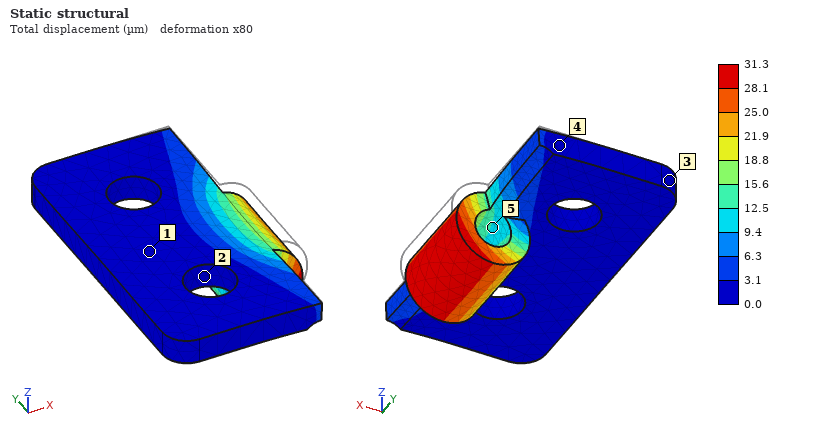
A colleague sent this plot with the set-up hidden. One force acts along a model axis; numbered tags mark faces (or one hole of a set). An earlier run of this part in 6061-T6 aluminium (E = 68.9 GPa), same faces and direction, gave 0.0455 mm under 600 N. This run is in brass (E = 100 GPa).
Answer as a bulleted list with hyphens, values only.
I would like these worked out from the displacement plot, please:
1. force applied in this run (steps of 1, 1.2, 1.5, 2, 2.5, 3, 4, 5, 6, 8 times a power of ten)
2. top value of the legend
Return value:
- 600 N
- 31.3 µm
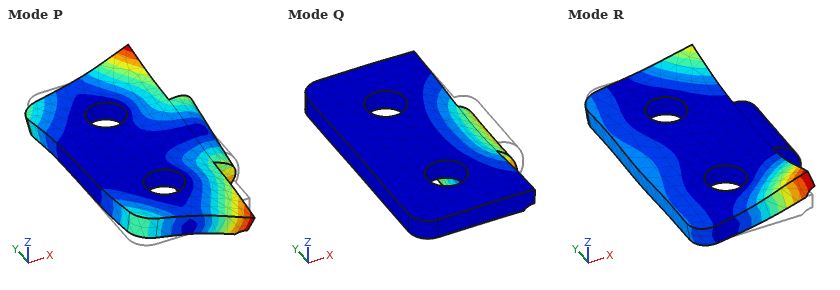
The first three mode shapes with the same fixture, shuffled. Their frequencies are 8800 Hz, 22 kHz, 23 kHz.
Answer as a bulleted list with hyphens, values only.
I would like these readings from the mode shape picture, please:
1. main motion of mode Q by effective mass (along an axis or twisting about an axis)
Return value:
- along Z
